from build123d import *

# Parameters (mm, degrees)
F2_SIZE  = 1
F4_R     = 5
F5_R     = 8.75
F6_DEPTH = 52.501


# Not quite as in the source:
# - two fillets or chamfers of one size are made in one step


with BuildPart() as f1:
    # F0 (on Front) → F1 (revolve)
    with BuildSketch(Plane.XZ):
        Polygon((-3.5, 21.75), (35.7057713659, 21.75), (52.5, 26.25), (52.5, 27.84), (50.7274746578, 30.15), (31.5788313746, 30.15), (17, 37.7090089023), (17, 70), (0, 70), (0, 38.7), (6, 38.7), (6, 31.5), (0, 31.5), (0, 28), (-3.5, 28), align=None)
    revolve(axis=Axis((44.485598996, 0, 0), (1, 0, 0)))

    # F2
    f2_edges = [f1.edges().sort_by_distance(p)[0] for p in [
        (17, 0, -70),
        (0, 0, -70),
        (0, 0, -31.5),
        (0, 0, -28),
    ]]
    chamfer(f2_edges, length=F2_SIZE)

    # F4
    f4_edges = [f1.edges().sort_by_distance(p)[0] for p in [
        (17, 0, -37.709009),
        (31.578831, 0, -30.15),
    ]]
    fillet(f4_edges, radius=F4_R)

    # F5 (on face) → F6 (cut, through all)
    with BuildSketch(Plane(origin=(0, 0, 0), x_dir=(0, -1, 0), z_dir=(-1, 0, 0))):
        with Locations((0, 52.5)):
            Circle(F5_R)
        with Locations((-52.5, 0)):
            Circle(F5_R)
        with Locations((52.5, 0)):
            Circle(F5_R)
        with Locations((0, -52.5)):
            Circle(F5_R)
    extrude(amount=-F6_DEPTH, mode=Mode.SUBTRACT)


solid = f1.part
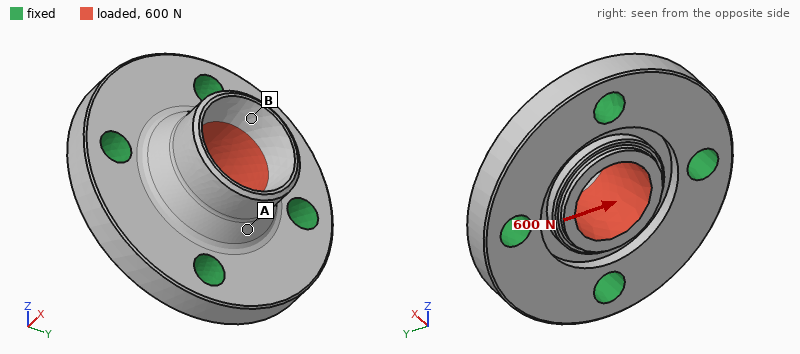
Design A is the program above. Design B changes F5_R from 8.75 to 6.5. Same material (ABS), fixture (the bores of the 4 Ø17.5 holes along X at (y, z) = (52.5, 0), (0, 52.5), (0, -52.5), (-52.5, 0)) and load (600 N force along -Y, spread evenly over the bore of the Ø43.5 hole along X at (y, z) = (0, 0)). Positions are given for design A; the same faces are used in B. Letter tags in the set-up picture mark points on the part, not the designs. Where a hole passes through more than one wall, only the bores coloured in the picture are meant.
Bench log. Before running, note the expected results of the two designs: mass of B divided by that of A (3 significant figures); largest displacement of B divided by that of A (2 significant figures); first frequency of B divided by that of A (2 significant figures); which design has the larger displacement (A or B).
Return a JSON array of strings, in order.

["1.03", "1.1", "0.88", "B"]
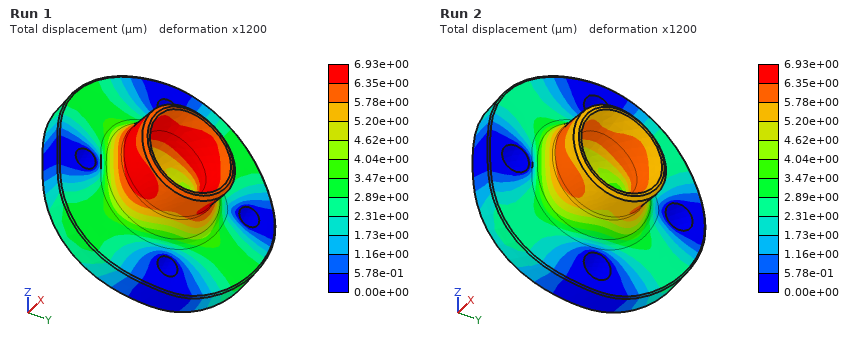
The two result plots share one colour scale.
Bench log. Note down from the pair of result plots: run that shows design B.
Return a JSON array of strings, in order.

["Run 1"]
